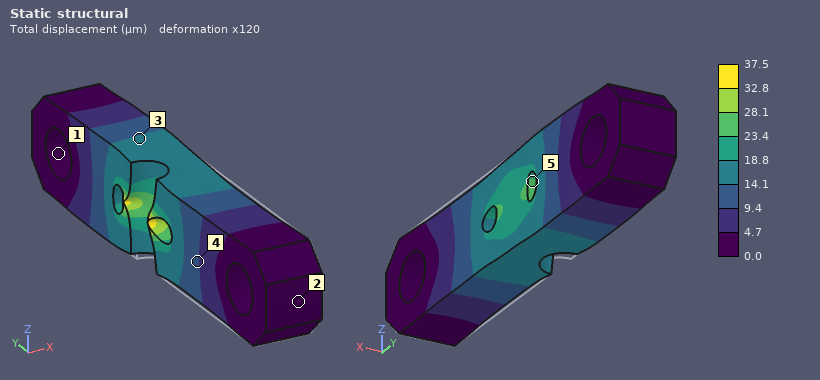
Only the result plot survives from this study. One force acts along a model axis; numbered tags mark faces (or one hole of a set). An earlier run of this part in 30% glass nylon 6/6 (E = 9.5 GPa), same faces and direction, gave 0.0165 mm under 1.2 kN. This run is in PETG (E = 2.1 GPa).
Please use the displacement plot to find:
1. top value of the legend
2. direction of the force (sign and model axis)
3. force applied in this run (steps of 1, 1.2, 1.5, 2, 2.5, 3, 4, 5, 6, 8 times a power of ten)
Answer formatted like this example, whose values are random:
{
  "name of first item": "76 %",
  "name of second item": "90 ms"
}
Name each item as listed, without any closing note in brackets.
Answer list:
{
  "top value of the legend": "37.5 µm",
  "direction of the force": "+Y",
  "force applied in this run": "600 N"
}
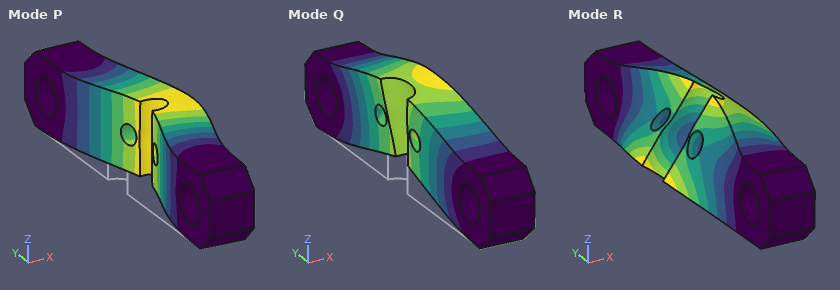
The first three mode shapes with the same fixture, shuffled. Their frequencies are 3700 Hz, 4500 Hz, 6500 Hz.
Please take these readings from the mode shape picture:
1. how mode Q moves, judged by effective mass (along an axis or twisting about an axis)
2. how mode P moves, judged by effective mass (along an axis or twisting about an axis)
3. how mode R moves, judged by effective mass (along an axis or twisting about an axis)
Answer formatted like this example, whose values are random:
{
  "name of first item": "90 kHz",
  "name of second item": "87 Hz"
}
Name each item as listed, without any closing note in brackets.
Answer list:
{
  "how mode Q moves, judged by effective mass": "along Z",
  "how mode P moves, judged by effective mass": "along X",
  "how mode R moves, judged by effective mass": "twisting about Y"
}
